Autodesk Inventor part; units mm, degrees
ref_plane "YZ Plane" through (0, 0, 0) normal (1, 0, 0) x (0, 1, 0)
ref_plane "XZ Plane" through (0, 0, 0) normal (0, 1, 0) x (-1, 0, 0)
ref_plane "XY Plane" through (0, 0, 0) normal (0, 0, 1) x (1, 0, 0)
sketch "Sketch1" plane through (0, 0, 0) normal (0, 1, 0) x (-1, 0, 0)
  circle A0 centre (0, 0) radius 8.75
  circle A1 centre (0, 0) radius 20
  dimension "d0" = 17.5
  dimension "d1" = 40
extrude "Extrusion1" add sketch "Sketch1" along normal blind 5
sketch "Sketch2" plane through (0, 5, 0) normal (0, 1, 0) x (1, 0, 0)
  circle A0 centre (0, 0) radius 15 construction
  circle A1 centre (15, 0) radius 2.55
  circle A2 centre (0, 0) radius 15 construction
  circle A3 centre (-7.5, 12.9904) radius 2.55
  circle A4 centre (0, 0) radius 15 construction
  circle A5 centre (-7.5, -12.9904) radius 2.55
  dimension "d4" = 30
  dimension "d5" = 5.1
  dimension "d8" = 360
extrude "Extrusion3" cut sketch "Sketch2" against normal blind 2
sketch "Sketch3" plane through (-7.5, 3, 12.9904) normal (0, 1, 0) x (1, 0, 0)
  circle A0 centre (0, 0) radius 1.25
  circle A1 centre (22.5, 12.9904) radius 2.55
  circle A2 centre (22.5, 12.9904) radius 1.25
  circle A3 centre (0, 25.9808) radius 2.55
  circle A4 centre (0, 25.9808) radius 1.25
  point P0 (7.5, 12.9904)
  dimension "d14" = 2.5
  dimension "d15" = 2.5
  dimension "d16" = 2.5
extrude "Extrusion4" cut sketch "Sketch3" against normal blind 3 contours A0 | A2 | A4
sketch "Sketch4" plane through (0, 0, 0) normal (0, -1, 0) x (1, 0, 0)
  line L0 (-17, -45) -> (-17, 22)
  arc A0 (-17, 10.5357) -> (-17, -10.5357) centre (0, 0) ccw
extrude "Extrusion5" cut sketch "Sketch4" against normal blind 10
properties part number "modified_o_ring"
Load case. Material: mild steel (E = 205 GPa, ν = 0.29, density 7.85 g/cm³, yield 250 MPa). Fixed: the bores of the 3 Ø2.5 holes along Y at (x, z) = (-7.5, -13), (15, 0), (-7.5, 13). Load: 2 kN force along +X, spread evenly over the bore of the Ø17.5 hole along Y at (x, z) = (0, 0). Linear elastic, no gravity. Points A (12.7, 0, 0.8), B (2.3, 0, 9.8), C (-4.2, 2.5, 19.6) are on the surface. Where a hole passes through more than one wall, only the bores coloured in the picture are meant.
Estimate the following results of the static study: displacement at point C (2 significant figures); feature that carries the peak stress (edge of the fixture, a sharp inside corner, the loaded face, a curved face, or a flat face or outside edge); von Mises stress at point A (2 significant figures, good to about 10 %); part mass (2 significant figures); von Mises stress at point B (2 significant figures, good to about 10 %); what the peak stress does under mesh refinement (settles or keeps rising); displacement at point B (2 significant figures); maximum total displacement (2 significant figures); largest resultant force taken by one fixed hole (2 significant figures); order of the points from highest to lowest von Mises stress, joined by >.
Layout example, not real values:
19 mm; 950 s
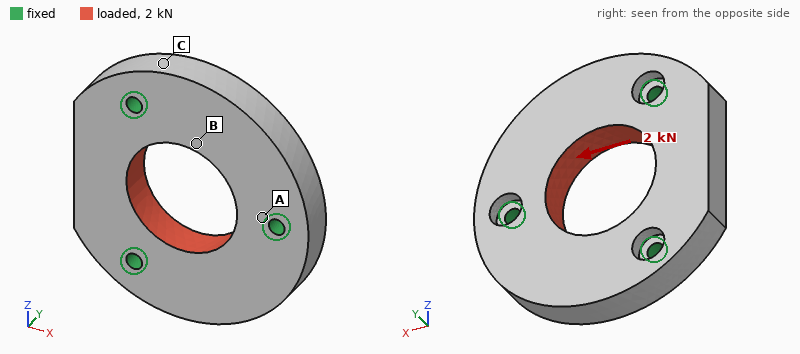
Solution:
0.57 µm; edge of the fixture; 17 MPa; 37 g; 10 MPa; keeps rising; 0.88 µm; 2.3 µm; 730 N; A > B > C
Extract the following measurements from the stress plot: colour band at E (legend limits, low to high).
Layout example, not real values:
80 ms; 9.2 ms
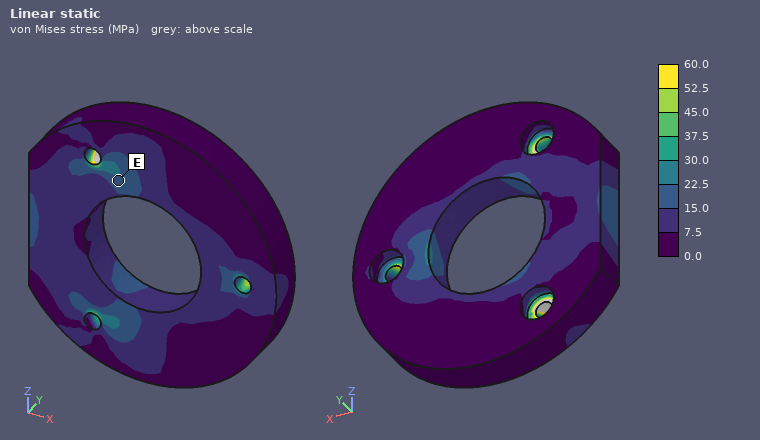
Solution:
15.0 to 22.5 MPa
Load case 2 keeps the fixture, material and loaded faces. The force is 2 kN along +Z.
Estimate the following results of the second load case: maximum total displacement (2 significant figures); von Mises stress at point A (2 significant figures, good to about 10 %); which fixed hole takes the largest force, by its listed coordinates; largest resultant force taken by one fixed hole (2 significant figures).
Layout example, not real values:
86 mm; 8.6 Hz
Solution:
2.0 µm; 19 MPa; (15, 0); 770 N
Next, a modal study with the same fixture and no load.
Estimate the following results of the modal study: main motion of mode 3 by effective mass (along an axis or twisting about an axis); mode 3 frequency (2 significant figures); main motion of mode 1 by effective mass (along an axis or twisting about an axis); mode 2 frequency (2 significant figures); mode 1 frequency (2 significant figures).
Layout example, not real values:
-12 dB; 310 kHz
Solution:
along Y; 21 kHz; twisting about X; 15 kHz; 14 kHz
